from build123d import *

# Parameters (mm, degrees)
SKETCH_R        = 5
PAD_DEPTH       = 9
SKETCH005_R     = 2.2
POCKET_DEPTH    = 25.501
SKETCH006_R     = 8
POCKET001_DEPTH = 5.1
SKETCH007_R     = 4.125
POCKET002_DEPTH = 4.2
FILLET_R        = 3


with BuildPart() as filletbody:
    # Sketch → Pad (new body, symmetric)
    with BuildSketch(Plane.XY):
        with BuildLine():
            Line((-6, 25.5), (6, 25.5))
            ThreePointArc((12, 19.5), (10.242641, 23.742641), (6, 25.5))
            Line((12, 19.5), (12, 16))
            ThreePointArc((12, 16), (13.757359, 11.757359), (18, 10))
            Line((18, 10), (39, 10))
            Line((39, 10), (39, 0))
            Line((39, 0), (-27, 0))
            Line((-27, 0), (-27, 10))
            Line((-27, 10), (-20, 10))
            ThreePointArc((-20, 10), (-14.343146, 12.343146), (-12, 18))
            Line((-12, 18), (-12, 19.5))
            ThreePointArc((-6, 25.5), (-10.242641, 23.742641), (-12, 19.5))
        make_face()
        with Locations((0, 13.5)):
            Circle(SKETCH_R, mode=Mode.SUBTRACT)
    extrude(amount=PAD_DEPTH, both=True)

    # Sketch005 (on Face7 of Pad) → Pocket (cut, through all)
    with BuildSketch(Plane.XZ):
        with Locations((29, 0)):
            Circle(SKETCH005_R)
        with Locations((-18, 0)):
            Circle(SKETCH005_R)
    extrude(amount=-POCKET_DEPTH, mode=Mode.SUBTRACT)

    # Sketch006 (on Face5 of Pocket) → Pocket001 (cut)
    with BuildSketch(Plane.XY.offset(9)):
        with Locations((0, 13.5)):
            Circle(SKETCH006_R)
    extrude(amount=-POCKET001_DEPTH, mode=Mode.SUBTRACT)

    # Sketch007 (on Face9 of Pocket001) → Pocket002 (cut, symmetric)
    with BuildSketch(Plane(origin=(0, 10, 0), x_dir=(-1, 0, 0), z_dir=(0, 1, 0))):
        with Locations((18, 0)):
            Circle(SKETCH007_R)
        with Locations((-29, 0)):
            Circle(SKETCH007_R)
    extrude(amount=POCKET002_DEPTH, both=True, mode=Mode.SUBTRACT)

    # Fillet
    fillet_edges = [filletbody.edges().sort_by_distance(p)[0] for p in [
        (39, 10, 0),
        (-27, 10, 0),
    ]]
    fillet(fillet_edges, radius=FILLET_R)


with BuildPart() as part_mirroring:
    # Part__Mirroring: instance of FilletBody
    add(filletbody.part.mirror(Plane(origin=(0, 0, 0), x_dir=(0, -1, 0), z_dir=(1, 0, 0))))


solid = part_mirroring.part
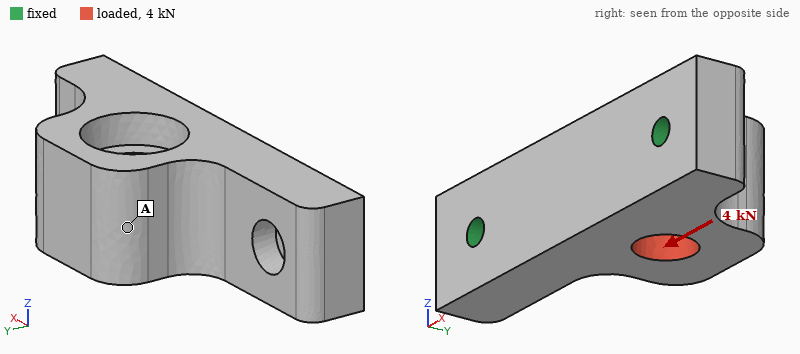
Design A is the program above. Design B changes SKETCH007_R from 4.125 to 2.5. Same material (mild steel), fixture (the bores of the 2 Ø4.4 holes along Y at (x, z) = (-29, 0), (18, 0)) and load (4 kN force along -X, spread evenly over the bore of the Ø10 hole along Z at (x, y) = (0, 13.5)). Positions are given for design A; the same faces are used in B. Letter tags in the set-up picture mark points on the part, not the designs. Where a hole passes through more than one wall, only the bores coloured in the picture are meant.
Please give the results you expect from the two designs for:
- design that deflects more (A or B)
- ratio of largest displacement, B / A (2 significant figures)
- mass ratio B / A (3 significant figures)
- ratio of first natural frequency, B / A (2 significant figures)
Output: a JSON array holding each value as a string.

["A", "0.92", "1.02", "1.1"]
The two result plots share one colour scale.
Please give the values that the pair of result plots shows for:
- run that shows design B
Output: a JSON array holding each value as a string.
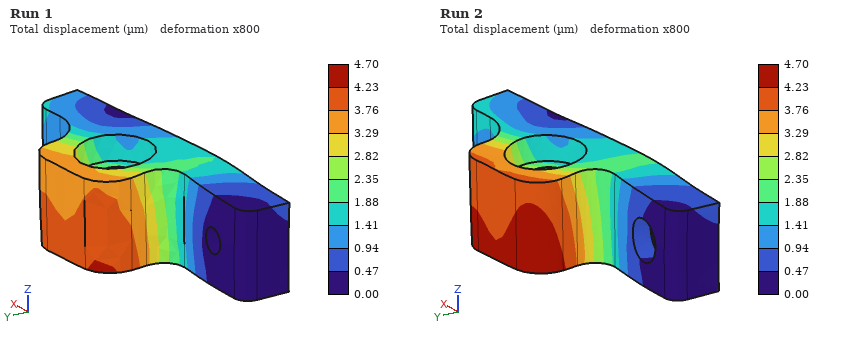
["Run 1"]
